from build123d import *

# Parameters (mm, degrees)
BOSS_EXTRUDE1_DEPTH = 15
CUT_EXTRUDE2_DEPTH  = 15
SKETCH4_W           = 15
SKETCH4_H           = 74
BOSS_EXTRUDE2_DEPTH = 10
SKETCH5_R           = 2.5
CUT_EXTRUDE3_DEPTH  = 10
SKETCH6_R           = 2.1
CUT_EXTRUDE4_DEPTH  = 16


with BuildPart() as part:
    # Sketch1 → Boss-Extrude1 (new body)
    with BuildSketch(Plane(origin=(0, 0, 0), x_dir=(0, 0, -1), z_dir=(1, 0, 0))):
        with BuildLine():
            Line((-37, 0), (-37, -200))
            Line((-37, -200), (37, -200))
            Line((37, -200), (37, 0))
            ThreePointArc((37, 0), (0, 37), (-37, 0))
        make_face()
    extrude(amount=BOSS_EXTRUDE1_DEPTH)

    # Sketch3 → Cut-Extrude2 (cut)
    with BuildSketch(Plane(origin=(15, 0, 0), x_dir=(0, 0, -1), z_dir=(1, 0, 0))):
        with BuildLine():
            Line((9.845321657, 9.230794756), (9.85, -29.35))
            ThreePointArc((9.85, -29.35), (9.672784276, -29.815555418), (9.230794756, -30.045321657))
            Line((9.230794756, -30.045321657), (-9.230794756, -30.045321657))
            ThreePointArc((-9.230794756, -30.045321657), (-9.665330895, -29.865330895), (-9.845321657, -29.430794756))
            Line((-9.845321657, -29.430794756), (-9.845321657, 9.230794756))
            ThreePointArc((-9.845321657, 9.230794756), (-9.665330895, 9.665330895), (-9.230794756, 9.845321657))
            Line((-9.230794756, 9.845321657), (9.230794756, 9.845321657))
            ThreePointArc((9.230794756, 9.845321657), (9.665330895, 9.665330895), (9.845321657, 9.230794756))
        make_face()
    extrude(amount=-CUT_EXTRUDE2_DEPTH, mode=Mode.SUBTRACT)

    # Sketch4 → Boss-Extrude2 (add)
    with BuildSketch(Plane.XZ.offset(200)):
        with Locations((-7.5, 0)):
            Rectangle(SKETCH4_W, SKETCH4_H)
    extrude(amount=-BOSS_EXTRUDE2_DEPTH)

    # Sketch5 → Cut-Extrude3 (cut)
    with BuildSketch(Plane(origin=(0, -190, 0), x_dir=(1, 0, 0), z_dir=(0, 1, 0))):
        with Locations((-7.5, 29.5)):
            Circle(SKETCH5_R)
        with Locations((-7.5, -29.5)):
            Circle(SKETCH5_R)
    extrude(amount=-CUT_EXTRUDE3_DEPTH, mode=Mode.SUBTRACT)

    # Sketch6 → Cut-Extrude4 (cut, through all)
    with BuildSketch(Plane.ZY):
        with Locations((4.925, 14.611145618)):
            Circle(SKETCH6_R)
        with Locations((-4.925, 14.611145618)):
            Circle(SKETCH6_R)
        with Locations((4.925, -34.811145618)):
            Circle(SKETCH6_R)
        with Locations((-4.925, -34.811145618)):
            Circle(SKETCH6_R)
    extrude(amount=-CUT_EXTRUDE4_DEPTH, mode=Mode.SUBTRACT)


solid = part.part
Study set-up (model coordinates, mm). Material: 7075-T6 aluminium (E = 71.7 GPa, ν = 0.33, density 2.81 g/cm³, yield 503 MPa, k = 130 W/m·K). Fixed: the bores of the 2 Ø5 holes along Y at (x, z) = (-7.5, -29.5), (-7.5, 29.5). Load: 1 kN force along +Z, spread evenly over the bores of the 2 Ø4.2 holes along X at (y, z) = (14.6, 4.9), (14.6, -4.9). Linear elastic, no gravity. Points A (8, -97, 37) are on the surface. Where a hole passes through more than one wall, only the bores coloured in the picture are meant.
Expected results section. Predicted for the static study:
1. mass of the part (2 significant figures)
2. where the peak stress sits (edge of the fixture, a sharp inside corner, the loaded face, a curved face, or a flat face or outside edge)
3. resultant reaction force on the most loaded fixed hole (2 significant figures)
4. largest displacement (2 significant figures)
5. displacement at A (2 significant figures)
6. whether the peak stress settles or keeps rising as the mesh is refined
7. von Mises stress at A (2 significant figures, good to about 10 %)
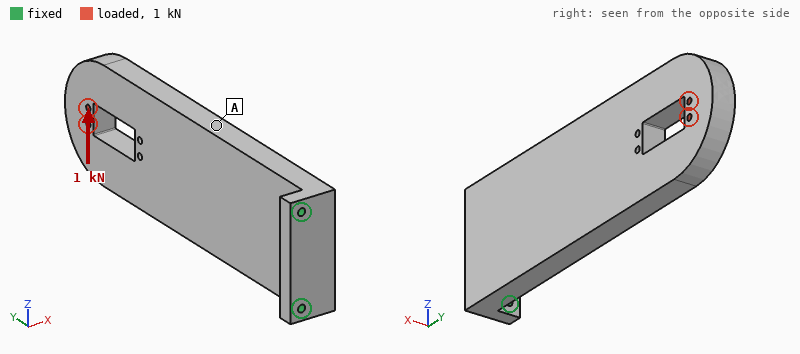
710 g
edge of the fixture
3.5 kN
0.26 mm
0.097 mm
keeps rising
8.2 MPa
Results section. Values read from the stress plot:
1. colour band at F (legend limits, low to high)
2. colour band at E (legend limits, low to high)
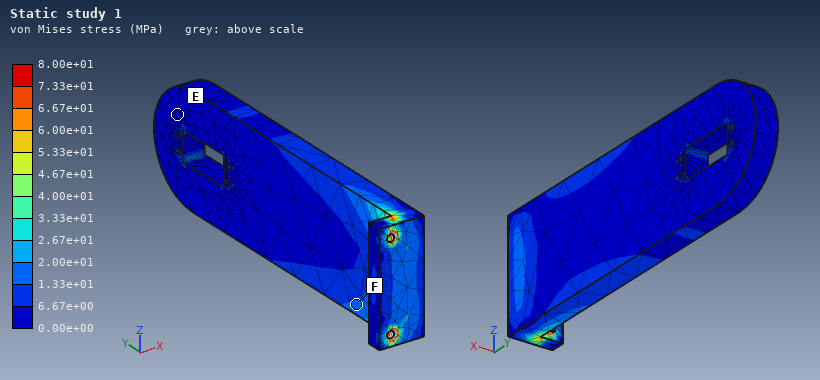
1.33e+01 to 2.00e+01 MPa
0.00e+00 to 6.67e+00 MPa
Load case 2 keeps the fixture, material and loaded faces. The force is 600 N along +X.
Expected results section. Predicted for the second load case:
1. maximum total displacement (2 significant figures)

2.7 mm
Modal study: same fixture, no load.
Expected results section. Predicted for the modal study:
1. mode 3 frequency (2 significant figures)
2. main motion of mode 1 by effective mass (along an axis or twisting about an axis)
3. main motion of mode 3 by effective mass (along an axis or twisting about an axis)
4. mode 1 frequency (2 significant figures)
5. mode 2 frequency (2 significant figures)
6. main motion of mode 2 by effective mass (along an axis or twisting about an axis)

1200 Hz
along X
along X
180 Hz
710 Hz
along Z
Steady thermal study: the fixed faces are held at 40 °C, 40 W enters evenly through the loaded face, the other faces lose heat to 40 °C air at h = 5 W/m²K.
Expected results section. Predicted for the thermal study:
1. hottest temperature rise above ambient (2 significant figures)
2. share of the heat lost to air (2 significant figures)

72 K
18 %
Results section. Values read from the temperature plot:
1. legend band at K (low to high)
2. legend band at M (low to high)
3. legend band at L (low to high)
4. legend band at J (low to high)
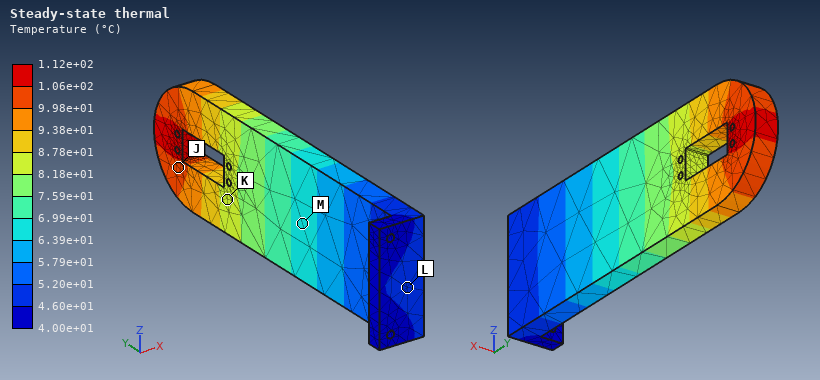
8.18e+01 to 8.78e+01 °C
6.39e+01 to 6.99e+01 °C
4.60e+01 to 5.20e+01 °C
9.98e+01 to 1.06e+02 °C
